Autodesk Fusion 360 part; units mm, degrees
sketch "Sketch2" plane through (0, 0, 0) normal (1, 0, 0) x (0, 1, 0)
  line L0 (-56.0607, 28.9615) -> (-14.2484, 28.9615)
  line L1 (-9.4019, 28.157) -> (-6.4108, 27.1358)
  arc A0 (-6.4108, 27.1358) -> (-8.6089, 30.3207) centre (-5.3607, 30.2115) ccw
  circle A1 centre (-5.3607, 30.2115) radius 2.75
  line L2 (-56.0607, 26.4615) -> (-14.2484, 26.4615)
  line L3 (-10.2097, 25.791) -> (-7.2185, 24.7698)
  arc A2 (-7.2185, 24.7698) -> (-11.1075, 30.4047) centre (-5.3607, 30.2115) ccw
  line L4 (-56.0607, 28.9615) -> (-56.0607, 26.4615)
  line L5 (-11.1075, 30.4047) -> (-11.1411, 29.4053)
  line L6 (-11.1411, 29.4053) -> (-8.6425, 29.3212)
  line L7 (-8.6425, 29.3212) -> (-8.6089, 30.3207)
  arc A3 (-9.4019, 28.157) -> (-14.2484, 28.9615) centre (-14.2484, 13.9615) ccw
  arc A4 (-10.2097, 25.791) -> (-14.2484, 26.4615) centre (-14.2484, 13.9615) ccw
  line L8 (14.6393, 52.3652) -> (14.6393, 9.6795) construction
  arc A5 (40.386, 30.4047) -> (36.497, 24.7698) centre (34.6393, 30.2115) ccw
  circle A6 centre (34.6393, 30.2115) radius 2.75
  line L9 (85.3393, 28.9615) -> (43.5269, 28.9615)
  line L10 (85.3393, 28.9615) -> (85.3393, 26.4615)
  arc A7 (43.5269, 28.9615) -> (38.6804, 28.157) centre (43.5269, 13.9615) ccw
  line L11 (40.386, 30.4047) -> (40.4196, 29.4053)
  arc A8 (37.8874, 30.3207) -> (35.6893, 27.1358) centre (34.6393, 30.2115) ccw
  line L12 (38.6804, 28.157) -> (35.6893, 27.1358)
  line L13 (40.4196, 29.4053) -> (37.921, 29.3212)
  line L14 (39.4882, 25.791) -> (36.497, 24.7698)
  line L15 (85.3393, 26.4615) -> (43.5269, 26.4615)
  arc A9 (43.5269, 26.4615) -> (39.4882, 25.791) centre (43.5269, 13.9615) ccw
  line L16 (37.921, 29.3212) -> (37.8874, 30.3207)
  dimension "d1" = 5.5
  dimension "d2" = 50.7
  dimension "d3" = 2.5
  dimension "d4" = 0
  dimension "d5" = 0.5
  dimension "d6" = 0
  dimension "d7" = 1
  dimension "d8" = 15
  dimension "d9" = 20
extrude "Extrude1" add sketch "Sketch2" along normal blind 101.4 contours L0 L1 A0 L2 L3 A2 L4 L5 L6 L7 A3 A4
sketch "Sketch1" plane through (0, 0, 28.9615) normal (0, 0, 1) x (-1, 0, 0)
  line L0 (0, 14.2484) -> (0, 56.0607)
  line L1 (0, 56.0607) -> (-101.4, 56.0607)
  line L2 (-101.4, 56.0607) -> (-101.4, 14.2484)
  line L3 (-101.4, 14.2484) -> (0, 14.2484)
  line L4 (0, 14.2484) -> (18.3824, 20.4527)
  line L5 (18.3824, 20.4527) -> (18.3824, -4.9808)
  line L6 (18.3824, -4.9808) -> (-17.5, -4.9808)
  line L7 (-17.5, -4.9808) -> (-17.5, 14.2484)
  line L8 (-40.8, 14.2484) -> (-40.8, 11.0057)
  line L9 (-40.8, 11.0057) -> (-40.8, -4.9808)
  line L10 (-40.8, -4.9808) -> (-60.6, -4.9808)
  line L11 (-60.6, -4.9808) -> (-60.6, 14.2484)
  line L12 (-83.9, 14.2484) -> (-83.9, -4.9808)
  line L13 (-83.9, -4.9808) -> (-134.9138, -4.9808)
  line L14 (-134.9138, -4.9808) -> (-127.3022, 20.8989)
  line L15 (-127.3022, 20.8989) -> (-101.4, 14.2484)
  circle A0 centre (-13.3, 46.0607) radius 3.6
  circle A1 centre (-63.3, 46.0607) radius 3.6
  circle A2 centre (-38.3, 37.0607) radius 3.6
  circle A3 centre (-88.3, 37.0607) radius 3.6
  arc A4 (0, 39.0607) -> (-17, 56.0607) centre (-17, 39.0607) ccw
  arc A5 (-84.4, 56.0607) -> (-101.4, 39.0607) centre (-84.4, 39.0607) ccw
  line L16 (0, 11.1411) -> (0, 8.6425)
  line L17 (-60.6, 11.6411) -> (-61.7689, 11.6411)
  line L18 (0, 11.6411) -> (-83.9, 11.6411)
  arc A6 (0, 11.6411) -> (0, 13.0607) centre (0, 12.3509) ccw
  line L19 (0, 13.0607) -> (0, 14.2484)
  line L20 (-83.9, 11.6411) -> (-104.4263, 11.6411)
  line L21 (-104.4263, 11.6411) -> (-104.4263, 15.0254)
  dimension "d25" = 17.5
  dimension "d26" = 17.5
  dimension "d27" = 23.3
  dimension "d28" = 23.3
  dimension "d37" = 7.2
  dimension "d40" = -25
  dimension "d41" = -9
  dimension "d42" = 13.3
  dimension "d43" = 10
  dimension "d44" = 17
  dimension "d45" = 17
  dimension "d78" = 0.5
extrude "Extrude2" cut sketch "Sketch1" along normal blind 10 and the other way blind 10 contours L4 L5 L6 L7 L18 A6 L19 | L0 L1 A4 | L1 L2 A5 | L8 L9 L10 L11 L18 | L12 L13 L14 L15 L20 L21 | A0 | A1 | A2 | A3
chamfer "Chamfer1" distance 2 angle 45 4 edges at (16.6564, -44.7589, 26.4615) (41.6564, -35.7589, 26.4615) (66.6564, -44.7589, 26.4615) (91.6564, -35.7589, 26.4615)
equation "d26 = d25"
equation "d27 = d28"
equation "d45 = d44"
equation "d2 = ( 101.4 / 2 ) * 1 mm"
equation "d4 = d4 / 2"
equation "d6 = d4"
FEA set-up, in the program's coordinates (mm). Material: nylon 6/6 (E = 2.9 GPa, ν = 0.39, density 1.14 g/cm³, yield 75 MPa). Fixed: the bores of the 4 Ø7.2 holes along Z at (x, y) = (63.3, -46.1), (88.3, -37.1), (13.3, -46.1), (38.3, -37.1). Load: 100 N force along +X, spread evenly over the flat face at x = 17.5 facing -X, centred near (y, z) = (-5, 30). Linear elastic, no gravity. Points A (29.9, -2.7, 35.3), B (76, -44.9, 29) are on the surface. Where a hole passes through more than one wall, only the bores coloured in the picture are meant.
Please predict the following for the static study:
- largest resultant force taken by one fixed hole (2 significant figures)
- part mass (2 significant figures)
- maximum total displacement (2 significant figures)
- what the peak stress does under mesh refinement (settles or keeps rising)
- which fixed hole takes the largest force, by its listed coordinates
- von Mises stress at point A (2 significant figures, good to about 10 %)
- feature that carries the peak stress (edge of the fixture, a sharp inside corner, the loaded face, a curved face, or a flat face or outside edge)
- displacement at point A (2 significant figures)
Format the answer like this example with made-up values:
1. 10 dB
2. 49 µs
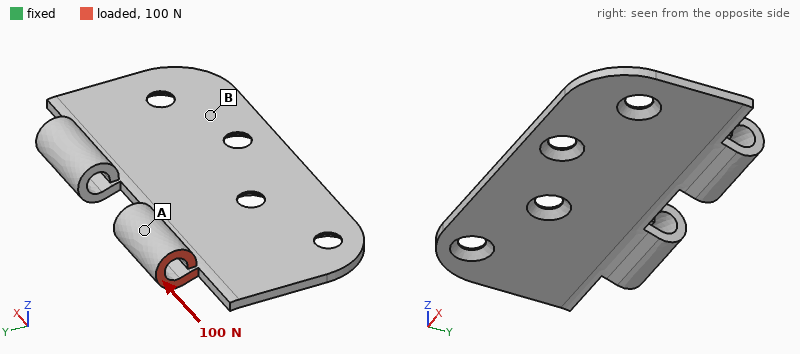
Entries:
1. 64 N
2. 16 g
3. 1.0 mm
4. keeps rising
5. (38.3, -37.1)
6. 4.0 MPa
7. edge of the fixture
8. 0.59 mm
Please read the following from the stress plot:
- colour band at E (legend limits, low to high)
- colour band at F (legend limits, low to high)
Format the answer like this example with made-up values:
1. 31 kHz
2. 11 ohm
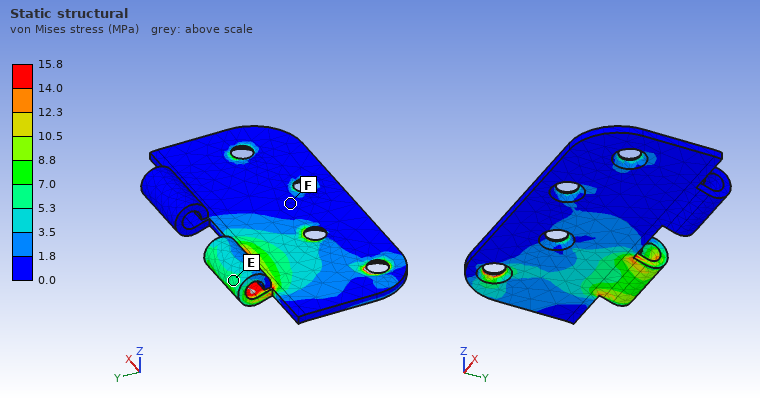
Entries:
1. 5.3 to 7.0 MPa
2. 0.0 to 1.8 MPa
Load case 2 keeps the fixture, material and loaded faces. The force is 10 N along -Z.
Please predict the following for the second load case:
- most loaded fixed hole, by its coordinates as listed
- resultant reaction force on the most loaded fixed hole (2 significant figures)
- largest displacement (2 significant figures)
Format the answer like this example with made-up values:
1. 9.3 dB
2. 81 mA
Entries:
1. (38.3, -37.1)
2. 22 N
3. 1.3 mm
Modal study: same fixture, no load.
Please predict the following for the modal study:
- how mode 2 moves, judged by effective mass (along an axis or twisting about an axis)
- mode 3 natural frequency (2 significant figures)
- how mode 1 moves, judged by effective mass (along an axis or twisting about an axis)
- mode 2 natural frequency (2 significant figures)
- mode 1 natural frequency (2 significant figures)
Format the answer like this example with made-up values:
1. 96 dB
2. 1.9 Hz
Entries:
1. twisting about Y
2. 870 Hz
3. along Z
4. 430 Hz
5. 330 Hz
